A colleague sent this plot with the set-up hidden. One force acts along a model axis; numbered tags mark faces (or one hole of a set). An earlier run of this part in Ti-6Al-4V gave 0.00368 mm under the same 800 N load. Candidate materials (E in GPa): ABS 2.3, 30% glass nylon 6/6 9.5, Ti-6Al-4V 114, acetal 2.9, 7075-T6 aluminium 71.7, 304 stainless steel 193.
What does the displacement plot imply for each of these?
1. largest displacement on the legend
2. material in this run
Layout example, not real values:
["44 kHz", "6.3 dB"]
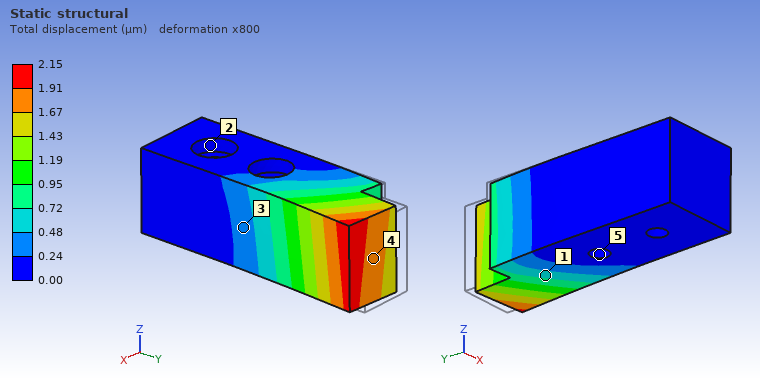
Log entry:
["2.15 µm", "304 stainless steel"]
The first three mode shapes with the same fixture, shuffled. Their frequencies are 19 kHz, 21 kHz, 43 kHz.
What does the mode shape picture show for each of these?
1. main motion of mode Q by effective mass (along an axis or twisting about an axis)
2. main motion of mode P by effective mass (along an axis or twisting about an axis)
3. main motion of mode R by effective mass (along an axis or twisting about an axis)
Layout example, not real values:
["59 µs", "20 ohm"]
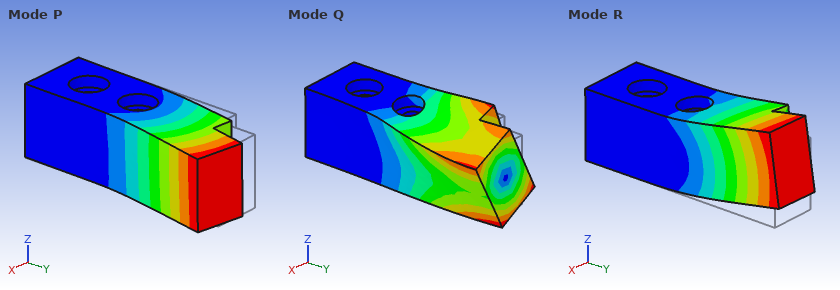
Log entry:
["twisting about Y", "along X", "along Z"]
